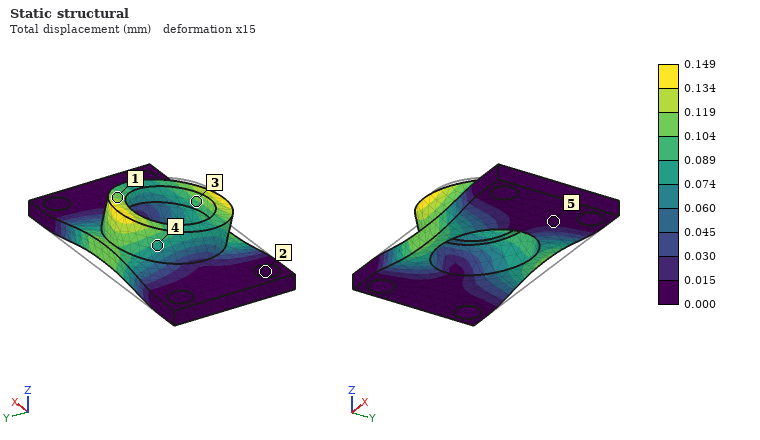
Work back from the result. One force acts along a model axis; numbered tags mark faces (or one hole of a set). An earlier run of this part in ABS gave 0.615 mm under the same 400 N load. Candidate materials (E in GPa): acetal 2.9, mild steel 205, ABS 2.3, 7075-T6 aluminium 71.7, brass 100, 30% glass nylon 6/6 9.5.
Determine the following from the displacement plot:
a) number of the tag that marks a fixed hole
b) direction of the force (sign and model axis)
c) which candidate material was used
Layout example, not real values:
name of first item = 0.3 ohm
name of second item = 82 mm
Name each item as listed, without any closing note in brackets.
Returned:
number of the tag that marks a fixed hole = 2
direction of the force = -Y
which candidate material was used = 30% glass nylon 6/6
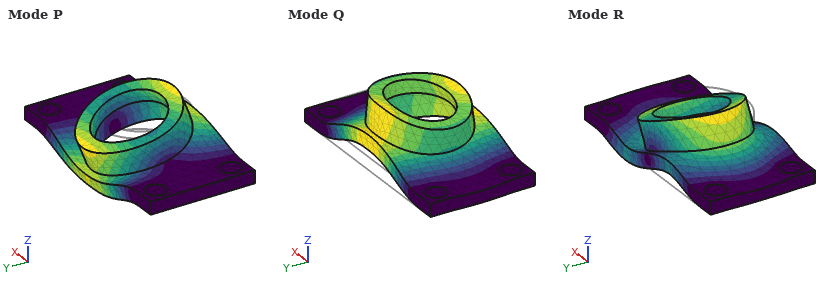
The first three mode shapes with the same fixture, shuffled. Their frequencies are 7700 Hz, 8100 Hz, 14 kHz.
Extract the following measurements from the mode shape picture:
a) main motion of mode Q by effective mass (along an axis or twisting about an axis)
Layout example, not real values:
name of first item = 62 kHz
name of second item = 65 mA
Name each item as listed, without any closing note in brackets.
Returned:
main motion of mode Q by effective mass = along Z
